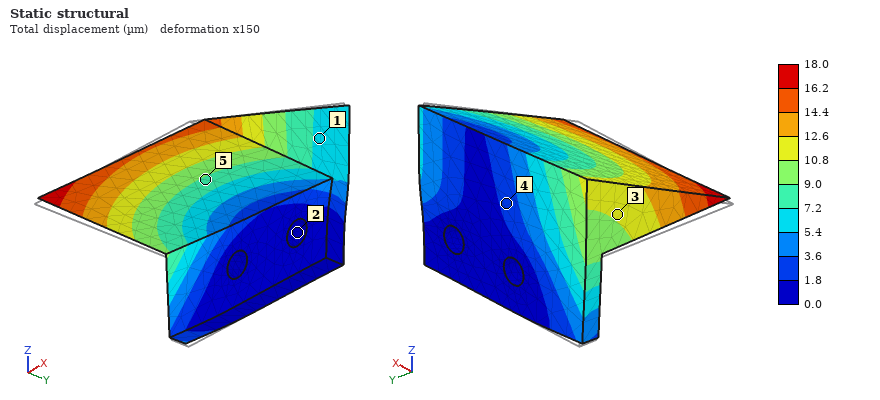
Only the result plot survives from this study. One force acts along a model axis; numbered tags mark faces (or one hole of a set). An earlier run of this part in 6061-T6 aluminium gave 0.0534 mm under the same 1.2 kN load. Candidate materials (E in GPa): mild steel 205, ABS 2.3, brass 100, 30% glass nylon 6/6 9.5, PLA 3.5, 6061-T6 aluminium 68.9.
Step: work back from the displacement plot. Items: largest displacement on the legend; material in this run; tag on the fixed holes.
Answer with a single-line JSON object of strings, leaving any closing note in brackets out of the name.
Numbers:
{"largest displacement on the legend": "18.0 µm", "material in this run": "mild steel", "tag on the fixed holes": "2"}
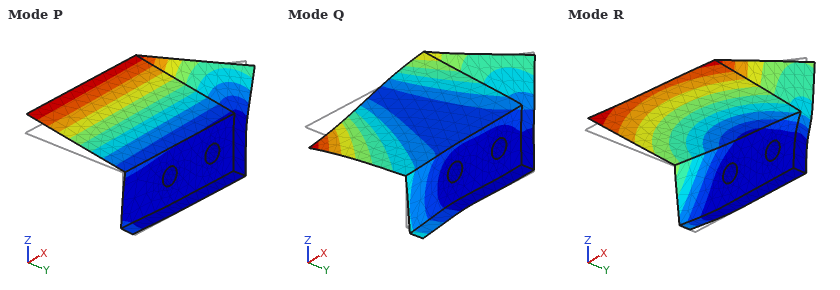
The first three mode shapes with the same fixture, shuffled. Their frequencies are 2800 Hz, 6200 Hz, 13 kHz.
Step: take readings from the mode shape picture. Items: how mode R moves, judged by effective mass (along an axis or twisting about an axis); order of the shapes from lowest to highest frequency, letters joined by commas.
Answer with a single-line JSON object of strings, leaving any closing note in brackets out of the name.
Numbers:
{"how mode R moves, judged by effective mass": "along X", "order of the shapes from lowest to highest frequency, letters joined by commas": "P, R, Q"}
